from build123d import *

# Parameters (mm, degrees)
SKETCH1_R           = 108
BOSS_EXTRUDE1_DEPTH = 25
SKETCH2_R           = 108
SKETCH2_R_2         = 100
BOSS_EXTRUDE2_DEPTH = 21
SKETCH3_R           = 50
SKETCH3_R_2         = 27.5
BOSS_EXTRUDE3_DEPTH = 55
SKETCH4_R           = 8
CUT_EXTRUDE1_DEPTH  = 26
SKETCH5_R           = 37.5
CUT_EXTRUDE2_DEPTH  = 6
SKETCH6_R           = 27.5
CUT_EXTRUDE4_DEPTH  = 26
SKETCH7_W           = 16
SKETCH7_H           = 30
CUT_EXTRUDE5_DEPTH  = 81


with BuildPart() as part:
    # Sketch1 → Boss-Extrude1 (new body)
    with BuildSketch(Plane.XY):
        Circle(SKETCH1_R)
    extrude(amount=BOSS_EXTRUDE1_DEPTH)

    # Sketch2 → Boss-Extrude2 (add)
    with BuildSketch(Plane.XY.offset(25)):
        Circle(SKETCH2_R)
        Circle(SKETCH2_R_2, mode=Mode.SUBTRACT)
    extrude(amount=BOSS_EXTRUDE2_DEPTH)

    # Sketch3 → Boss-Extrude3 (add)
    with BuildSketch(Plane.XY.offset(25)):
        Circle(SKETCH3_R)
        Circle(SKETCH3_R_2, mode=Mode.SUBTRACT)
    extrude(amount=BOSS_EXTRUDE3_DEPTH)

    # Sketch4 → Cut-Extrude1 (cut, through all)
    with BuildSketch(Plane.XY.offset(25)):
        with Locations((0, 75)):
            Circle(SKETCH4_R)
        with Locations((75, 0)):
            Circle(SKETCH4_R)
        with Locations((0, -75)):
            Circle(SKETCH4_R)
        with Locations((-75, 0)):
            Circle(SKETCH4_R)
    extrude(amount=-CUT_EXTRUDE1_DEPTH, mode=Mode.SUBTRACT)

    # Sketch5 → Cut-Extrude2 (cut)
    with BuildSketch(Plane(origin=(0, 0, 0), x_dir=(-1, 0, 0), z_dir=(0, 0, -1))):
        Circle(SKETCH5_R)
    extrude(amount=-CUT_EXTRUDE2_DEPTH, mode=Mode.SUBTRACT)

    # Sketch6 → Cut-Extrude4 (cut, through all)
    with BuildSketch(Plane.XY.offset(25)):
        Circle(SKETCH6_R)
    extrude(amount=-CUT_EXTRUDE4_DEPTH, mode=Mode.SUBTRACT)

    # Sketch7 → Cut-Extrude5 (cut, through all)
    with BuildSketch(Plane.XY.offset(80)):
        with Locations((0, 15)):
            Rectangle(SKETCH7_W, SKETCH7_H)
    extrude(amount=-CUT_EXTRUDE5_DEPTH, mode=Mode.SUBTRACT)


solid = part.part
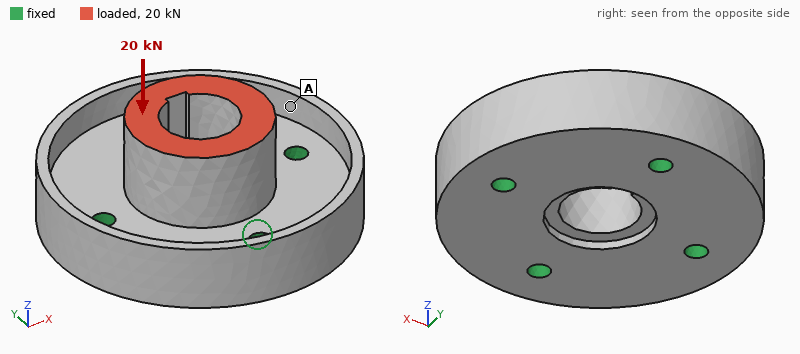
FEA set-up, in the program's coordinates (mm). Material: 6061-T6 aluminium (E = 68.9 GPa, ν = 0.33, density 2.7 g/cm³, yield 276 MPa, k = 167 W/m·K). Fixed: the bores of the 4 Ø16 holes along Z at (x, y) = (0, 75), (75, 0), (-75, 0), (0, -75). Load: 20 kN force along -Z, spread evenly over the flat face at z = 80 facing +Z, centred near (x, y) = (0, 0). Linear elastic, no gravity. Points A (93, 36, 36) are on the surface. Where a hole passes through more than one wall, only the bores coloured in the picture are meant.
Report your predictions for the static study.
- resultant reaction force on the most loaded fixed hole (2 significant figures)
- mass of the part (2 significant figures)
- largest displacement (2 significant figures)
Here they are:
5.4 kN
3.3 kg
11 µm
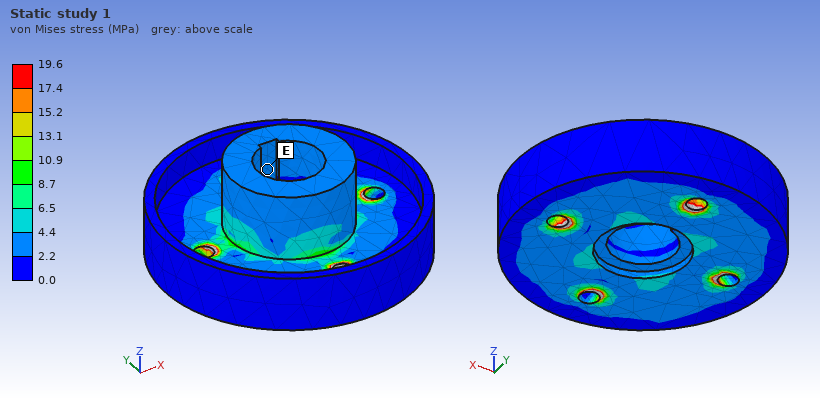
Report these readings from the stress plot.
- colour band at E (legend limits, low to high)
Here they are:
2.2 to 4.4 MPa
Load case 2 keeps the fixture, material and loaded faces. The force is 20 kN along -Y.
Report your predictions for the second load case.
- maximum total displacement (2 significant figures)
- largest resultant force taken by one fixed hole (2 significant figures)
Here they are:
44 µm
12 kN
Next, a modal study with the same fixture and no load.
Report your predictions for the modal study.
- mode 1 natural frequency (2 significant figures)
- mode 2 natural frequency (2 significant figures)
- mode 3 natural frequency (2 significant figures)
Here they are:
4800 Hz
5200 Hz
5200 Hz
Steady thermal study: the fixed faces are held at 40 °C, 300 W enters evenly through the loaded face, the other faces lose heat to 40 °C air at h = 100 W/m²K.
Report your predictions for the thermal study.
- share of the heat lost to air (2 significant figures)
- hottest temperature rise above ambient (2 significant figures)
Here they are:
24 %
25 K
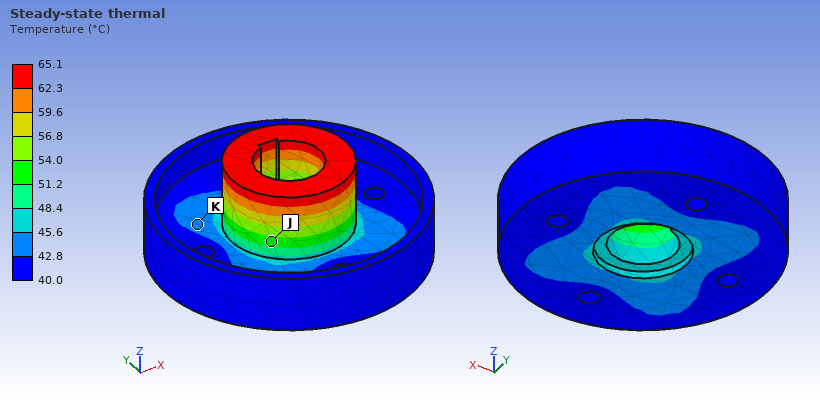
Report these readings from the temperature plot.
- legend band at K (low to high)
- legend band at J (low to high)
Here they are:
42.8 to 45.6 °C
51.2 to 54.0 °C
